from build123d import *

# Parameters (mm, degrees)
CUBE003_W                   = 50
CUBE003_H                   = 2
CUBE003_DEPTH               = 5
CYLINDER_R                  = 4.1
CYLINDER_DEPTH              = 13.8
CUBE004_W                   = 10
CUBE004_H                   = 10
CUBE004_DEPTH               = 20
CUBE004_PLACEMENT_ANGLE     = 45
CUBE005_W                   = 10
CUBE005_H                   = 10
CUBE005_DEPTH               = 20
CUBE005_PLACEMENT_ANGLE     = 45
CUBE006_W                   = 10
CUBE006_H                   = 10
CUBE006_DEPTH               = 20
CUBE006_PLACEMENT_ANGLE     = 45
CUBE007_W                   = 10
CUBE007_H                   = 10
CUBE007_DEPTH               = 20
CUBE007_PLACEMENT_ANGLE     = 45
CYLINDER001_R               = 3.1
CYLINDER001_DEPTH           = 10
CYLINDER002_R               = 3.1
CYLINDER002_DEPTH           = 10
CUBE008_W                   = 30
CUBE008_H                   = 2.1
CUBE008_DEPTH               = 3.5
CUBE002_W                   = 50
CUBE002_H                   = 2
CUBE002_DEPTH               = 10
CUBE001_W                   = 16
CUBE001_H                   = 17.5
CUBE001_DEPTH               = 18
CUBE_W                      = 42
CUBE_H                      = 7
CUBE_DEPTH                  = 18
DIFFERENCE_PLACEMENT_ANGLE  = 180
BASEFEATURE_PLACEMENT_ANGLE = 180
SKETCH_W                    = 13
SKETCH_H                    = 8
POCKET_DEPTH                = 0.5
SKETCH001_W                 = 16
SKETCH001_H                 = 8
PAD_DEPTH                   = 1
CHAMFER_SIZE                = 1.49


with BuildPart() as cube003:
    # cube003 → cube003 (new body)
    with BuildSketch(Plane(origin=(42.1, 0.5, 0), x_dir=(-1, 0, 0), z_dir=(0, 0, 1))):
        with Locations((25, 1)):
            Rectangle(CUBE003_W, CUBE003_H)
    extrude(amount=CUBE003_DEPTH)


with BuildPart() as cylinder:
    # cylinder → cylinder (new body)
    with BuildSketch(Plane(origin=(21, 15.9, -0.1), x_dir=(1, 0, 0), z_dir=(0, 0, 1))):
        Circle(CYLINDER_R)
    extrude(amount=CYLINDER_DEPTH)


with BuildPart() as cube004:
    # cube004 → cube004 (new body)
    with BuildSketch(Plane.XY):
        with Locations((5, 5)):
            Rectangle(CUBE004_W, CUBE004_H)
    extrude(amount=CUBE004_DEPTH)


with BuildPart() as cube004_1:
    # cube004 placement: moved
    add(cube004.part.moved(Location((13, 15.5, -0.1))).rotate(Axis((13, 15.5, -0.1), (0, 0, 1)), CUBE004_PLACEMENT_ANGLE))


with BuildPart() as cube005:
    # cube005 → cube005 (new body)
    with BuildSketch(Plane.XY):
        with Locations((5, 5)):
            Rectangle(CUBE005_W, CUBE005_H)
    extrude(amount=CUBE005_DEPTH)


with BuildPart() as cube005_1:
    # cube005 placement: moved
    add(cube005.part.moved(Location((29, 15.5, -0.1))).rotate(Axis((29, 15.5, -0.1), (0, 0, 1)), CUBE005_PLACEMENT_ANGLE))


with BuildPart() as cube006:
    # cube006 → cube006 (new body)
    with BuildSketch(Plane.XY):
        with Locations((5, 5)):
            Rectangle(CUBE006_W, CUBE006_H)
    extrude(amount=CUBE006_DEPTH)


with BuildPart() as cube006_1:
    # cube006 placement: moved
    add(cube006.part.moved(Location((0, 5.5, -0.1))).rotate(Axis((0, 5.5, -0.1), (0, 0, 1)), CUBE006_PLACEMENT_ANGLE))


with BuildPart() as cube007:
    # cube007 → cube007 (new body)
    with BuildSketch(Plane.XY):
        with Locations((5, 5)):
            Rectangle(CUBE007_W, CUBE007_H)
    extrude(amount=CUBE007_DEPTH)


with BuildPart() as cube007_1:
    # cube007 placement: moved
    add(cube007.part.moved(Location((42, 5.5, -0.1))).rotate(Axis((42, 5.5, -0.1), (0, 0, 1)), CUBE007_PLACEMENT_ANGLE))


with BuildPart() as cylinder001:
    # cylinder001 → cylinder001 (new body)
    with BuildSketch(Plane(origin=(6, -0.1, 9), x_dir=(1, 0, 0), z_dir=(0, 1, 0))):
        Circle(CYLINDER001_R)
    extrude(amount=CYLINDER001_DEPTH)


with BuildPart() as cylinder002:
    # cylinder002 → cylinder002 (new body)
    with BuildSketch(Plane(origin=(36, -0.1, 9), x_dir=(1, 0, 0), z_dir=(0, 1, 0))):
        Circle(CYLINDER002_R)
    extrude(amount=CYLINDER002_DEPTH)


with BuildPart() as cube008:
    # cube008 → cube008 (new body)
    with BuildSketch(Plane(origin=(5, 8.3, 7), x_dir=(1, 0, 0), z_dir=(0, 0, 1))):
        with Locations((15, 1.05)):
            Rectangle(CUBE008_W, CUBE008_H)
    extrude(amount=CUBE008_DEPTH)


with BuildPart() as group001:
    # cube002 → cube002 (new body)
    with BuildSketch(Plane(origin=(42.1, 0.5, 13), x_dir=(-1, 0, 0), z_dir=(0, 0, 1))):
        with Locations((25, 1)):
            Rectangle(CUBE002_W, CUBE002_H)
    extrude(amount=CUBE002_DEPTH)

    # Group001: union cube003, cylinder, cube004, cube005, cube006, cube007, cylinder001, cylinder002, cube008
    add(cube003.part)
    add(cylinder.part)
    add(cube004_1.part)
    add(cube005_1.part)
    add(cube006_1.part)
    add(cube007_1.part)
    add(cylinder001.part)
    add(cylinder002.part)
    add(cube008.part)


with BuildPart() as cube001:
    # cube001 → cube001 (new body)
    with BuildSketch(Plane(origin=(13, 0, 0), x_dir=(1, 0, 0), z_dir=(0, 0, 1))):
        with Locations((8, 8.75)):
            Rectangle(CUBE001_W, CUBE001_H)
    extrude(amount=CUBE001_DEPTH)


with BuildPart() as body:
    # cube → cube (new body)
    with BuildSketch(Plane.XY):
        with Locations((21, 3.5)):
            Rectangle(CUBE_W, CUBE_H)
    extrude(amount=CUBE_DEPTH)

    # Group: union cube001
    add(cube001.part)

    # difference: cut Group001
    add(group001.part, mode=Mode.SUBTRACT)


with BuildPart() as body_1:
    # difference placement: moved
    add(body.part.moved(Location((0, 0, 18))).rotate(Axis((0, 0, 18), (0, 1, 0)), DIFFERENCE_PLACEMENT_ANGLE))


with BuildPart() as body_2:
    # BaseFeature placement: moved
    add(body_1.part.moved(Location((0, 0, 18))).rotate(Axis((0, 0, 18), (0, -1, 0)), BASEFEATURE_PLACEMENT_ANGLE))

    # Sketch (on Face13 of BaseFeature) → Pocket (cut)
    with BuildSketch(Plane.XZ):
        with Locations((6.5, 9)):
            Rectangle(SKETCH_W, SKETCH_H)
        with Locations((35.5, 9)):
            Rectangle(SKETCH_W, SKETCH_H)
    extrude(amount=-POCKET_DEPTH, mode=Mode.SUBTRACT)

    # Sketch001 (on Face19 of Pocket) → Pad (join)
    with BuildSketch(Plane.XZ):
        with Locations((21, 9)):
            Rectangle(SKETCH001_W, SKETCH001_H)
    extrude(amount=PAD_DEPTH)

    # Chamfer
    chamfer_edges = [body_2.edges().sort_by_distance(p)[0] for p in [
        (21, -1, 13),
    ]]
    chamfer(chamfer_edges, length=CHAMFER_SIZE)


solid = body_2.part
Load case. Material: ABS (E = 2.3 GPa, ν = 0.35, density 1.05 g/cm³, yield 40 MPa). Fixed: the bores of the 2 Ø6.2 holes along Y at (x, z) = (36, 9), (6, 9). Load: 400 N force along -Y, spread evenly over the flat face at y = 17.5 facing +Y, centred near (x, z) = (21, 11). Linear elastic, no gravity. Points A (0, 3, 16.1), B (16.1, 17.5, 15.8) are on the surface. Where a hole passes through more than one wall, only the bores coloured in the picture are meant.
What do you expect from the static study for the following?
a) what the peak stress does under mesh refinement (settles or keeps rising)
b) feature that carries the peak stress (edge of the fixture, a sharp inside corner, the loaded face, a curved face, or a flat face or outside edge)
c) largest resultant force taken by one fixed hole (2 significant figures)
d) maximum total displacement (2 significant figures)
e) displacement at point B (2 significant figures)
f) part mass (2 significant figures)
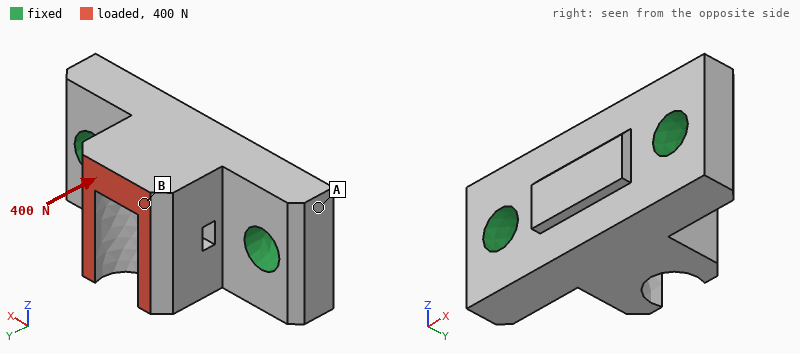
keeps rising
edge of the fixture
210 N
76 µm
66 µm
7.3 g
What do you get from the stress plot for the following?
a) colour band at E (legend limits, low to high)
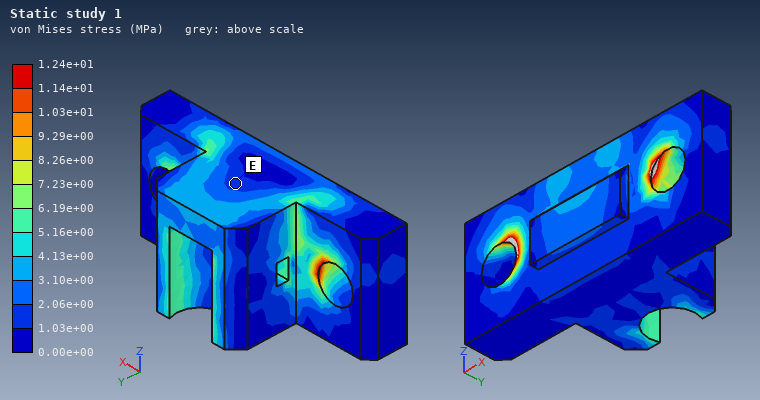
1.03e+00 to 2.06e+00 MPa
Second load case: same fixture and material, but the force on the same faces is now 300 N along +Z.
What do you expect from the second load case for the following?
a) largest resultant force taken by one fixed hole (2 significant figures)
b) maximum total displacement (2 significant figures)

150 N
0.27 mm
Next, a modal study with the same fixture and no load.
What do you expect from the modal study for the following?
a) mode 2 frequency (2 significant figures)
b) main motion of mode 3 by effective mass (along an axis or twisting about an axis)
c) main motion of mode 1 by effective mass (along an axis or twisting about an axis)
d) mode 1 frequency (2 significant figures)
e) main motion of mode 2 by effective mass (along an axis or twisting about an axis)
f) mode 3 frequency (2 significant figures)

8200 Hz
along X
along Z
5100 Hz
along Y
9900 Hz
